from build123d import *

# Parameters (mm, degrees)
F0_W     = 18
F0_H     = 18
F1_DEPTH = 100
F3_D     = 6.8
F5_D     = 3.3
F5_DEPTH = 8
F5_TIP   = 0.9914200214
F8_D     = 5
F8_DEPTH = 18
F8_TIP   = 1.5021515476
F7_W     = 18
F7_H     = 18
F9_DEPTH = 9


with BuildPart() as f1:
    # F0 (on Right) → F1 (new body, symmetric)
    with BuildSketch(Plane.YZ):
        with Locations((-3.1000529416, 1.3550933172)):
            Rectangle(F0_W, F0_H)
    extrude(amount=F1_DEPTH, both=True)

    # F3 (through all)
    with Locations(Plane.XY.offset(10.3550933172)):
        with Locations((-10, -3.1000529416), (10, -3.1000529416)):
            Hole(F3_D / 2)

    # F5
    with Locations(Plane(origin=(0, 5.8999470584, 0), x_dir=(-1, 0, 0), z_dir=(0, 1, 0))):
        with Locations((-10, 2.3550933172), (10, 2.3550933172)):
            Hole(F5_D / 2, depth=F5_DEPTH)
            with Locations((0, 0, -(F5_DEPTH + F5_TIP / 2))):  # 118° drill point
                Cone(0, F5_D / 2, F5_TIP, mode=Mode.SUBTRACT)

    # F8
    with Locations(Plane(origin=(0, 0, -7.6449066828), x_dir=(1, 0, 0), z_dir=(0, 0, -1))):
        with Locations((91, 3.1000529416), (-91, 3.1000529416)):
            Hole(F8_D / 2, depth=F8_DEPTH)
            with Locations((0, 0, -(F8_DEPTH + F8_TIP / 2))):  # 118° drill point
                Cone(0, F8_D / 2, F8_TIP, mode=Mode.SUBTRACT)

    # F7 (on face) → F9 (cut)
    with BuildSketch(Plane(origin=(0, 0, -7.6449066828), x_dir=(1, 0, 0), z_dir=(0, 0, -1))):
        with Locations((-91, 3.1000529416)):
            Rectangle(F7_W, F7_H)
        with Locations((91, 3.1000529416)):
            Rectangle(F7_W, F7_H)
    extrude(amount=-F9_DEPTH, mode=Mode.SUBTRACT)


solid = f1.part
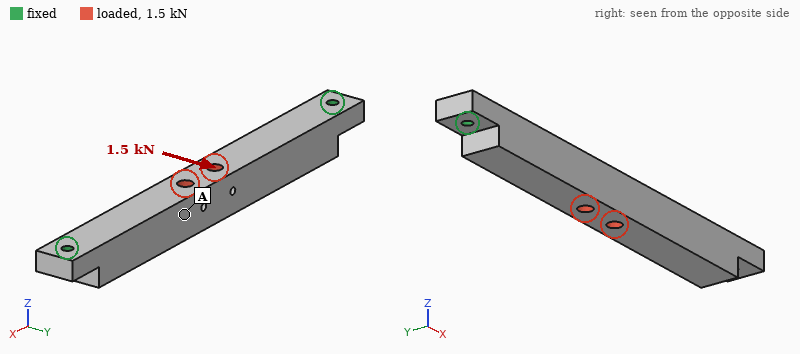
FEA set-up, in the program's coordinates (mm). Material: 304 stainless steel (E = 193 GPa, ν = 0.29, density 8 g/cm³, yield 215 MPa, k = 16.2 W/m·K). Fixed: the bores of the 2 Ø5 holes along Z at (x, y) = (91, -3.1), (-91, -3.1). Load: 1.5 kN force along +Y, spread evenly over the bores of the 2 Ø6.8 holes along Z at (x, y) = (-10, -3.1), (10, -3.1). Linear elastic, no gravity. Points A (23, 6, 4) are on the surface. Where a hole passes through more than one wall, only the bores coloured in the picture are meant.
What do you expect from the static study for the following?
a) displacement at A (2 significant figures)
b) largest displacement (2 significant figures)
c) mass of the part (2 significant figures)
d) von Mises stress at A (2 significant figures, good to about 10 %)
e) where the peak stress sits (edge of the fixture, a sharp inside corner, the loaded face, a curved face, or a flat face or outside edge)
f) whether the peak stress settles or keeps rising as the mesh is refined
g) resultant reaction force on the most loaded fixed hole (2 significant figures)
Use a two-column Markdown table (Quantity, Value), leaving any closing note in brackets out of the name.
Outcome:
| Quantity | Value |
|---|---|
| displacement at A | 48 µm |
| largest displacement | 56 µm |
| mass of the part | 460 g |
| von Mises stress at A | 27 MPa |
| where the peak stress sits | edge of the fixture |
| whether the peak stress settles or keeps rising as the mesh is refined | keeps rising |
| resultant reaction force on the most loaded fixed hole | 750 N |
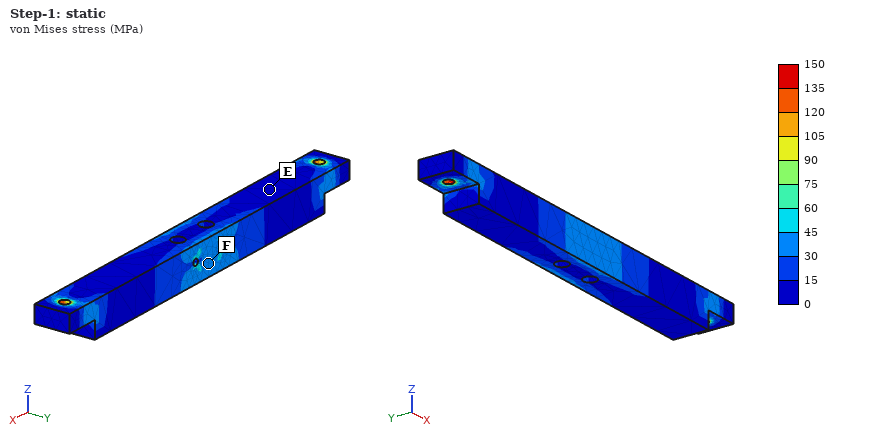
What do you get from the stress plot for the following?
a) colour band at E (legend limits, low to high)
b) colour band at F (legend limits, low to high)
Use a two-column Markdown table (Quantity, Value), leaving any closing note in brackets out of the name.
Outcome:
| Quantity | Value |
|---|---|
| colour band at E | 0 to 15 MPa |
| colour band at F | 30 to 45 MPa |
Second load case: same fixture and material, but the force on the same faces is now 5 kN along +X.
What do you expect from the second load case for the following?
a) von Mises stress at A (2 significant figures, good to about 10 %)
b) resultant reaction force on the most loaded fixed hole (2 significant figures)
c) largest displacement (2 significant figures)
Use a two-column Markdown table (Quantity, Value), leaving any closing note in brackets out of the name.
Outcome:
| Quantity | Value |
|---|---|
| von Mises stress at A | 8.4 MPa |
| resultant reaction force on the most loaded fixed hole | 2.5 kN |
| largest displacement | 5.5 µm |
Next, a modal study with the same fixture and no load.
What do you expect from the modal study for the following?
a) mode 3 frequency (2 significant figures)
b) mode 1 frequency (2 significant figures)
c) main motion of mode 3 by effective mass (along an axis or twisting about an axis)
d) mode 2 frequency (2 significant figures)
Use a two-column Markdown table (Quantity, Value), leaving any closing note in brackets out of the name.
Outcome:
| Quantity | Value |
|---|---|
| mode 3 frequency | 5200 Hz |
| mode 1 frequency | 1800 Hz |
| main motion of mode 3 by effective mass | twisting about Z |
| mode 2 frequency | 1800 Hz |
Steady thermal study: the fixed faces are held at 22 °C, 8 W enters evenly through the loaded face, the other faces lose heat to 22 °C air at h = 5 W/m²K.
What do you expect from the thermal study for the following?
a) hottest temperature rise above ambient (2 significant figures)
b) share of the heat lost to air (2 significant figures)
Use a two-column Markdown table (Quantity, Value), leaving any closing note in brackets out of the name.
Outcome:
| Quantity | Value |
|---|---|
| hottest temperature rise above ambient | 60 K |
| share of the heat lost to air | 28 % |
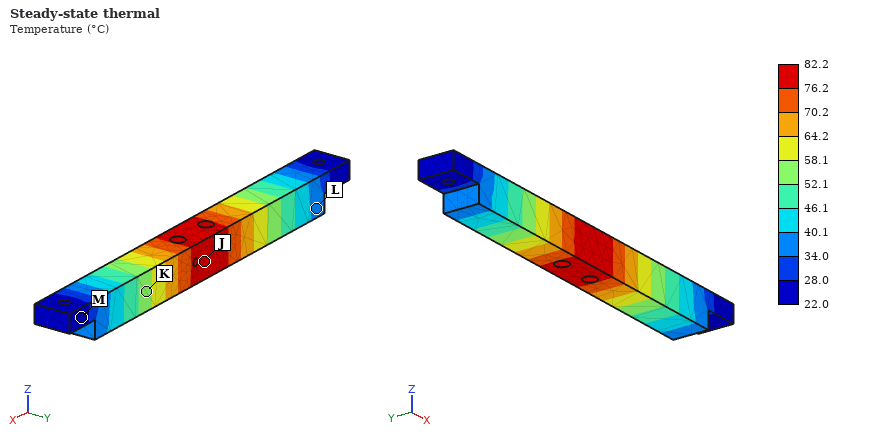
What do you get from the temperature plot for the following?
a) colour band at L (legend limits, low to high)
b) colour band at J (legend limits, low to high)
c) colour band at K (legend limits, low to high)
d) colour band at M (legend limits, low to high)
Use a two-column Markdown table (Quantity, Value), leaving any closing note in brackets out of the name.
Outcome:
| Quantity | Value |
|---|---|
| colour band at L | 34.0 to 40.1 °C |
| colour band at J | 76.2 to 82.2 °C |
| colour band at K | 52.1 to 58.1 °C |
| colour band at M | 22.0 to 28.0 °C |
